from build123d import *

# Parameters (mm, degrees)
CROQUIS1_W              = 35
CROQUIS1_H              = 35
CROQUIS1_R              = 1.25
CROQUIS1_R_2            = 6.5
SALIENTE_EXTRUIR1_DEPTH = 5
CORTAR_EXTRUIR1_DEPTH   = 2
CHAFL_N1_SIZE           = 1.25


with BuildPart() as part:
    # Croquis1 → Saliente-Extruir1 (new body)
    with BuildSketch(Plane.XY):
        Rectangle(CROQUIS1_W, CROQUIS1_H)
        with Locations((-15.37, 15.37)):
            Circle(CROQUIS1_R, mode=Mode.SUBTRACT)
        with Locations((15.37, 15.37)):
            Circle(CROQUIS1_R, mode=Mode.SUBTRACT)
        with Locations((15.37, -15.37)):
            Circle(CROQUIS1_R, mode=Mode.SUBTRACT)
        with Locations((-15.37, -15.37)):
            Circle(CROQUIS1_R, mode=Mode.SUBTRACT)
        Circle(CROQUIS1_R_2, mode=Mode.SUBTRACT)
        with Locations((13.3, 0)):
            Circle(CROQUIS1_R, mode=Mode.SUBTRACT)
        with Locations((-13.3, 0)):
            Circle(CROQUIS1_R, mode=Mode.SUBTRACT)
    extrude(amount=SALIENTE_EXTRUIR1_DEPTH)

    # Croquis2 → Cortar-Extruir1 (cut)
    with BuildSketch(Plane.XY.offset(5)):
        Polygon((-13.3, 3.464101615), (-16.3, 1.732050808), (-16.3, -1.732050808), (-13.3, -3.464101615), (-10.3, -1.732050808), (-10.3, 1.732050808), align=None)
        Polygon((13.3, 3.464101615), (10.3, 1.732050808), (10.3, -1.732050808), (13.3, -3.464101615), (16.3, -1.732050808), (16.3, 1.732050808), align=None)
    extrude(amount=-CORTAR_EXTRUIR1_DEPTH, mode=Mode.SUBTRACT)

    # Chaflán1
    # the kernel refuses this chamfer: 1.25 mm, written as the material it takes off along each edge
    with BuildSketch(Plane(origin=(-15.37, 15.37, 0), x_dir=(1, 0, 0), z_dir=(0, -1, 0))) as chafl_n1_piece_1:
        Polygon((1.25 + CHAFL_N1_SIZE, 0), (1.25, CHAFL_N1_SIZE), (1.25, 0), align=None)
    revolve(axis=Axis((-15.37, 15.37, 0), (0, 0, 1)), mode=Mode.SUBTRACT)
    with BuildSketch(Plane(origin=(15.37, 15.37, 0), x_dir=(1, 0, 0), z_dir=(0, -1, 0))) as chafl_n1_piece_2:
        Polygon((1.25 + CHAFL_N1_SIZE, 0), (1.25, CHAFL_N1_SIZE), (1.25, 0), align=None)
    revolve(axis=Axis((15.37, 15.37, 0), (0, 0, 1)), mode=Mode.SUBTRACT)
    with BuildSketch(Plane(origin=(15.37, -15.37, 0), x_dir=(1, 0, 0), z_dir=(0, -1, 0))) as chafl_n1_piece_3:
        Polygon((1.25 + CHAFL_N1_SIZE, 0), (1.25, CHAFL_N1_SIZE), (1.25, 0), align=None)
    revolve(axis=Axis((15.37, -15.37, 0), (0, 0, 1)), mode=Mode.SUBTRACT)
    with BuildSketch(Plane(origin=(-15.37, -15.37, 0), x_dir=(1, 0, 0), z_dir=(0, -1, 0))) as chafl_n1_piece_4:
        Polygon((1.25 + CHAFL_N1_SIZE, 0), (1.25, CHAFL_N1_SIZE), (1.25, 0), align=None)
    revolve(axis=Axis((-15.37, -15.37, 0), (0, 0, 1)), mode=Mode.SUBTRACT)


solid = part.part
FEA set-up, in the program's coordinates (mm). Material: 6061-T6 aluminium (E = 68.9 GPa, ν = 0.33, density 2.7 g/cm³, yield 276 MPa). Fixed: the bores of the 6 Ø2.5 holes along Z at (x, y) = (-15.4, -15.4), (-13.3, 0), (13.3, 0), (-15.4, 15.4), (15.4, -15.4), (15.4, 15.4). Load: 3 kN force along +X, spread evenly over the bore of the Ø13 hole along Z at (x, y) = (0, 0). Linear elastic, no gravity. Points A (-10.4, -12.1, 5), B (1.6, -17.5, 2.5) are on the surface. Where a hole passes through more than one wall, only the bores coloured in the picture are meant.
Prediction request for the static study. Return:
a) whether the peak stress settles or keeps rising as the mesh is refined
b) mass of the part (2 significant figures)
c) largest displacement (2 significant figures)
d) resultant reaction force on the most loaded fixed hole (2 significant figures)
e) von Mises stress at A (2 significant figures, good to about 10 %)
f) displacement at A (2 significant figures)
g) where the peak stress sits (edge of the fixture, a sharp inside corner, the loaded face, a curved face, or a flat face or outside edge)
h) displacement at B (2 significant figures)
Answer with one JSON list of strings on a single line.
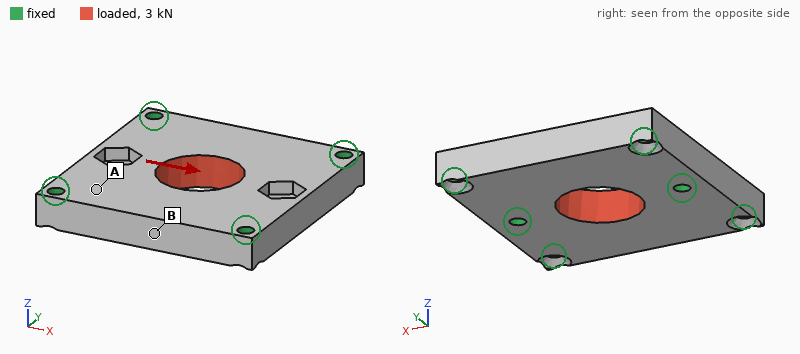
["keeps rising", "14 g", "3.5 µm", "780 N", "13 MPa", "1.2 µm", "edge of the fixture", "0.90 µm"]
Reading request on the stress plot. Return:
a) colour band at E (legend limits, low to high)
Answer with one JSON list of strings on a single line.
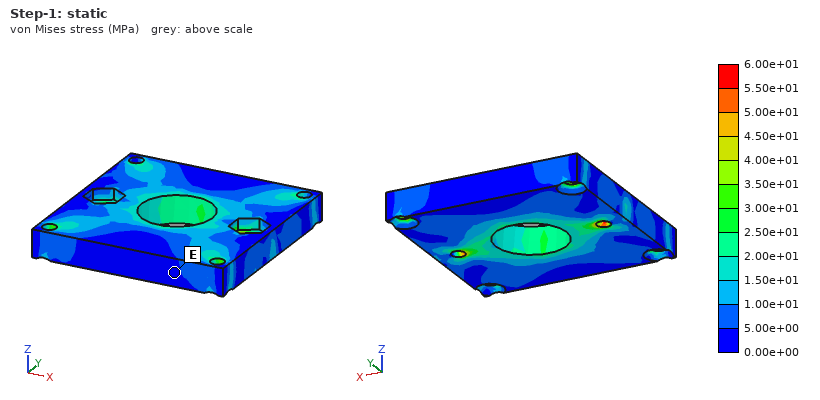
["0.00e+00 to 5.00e+00 MPa"]
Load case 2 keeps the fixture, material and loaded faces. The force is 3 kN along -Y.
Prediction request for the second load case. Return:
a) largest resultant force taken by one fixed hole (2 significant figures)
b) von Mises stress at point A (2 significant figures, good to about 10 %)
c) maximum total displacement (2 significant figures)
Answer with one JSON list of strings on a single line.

["750 N", "17 MPa", "5.8 µm"]
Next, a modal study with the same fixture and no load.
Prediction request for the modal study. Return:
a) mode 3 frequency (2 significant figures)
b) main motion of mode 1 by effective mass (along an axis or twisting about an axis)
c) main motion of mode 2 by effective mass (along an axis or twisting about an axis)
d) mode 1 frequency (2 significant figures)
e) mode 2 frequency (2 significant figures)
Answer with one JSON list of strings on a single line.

["42 kHz", "along Z", "twisting about X", "21 kHz", "23 kHz"]
